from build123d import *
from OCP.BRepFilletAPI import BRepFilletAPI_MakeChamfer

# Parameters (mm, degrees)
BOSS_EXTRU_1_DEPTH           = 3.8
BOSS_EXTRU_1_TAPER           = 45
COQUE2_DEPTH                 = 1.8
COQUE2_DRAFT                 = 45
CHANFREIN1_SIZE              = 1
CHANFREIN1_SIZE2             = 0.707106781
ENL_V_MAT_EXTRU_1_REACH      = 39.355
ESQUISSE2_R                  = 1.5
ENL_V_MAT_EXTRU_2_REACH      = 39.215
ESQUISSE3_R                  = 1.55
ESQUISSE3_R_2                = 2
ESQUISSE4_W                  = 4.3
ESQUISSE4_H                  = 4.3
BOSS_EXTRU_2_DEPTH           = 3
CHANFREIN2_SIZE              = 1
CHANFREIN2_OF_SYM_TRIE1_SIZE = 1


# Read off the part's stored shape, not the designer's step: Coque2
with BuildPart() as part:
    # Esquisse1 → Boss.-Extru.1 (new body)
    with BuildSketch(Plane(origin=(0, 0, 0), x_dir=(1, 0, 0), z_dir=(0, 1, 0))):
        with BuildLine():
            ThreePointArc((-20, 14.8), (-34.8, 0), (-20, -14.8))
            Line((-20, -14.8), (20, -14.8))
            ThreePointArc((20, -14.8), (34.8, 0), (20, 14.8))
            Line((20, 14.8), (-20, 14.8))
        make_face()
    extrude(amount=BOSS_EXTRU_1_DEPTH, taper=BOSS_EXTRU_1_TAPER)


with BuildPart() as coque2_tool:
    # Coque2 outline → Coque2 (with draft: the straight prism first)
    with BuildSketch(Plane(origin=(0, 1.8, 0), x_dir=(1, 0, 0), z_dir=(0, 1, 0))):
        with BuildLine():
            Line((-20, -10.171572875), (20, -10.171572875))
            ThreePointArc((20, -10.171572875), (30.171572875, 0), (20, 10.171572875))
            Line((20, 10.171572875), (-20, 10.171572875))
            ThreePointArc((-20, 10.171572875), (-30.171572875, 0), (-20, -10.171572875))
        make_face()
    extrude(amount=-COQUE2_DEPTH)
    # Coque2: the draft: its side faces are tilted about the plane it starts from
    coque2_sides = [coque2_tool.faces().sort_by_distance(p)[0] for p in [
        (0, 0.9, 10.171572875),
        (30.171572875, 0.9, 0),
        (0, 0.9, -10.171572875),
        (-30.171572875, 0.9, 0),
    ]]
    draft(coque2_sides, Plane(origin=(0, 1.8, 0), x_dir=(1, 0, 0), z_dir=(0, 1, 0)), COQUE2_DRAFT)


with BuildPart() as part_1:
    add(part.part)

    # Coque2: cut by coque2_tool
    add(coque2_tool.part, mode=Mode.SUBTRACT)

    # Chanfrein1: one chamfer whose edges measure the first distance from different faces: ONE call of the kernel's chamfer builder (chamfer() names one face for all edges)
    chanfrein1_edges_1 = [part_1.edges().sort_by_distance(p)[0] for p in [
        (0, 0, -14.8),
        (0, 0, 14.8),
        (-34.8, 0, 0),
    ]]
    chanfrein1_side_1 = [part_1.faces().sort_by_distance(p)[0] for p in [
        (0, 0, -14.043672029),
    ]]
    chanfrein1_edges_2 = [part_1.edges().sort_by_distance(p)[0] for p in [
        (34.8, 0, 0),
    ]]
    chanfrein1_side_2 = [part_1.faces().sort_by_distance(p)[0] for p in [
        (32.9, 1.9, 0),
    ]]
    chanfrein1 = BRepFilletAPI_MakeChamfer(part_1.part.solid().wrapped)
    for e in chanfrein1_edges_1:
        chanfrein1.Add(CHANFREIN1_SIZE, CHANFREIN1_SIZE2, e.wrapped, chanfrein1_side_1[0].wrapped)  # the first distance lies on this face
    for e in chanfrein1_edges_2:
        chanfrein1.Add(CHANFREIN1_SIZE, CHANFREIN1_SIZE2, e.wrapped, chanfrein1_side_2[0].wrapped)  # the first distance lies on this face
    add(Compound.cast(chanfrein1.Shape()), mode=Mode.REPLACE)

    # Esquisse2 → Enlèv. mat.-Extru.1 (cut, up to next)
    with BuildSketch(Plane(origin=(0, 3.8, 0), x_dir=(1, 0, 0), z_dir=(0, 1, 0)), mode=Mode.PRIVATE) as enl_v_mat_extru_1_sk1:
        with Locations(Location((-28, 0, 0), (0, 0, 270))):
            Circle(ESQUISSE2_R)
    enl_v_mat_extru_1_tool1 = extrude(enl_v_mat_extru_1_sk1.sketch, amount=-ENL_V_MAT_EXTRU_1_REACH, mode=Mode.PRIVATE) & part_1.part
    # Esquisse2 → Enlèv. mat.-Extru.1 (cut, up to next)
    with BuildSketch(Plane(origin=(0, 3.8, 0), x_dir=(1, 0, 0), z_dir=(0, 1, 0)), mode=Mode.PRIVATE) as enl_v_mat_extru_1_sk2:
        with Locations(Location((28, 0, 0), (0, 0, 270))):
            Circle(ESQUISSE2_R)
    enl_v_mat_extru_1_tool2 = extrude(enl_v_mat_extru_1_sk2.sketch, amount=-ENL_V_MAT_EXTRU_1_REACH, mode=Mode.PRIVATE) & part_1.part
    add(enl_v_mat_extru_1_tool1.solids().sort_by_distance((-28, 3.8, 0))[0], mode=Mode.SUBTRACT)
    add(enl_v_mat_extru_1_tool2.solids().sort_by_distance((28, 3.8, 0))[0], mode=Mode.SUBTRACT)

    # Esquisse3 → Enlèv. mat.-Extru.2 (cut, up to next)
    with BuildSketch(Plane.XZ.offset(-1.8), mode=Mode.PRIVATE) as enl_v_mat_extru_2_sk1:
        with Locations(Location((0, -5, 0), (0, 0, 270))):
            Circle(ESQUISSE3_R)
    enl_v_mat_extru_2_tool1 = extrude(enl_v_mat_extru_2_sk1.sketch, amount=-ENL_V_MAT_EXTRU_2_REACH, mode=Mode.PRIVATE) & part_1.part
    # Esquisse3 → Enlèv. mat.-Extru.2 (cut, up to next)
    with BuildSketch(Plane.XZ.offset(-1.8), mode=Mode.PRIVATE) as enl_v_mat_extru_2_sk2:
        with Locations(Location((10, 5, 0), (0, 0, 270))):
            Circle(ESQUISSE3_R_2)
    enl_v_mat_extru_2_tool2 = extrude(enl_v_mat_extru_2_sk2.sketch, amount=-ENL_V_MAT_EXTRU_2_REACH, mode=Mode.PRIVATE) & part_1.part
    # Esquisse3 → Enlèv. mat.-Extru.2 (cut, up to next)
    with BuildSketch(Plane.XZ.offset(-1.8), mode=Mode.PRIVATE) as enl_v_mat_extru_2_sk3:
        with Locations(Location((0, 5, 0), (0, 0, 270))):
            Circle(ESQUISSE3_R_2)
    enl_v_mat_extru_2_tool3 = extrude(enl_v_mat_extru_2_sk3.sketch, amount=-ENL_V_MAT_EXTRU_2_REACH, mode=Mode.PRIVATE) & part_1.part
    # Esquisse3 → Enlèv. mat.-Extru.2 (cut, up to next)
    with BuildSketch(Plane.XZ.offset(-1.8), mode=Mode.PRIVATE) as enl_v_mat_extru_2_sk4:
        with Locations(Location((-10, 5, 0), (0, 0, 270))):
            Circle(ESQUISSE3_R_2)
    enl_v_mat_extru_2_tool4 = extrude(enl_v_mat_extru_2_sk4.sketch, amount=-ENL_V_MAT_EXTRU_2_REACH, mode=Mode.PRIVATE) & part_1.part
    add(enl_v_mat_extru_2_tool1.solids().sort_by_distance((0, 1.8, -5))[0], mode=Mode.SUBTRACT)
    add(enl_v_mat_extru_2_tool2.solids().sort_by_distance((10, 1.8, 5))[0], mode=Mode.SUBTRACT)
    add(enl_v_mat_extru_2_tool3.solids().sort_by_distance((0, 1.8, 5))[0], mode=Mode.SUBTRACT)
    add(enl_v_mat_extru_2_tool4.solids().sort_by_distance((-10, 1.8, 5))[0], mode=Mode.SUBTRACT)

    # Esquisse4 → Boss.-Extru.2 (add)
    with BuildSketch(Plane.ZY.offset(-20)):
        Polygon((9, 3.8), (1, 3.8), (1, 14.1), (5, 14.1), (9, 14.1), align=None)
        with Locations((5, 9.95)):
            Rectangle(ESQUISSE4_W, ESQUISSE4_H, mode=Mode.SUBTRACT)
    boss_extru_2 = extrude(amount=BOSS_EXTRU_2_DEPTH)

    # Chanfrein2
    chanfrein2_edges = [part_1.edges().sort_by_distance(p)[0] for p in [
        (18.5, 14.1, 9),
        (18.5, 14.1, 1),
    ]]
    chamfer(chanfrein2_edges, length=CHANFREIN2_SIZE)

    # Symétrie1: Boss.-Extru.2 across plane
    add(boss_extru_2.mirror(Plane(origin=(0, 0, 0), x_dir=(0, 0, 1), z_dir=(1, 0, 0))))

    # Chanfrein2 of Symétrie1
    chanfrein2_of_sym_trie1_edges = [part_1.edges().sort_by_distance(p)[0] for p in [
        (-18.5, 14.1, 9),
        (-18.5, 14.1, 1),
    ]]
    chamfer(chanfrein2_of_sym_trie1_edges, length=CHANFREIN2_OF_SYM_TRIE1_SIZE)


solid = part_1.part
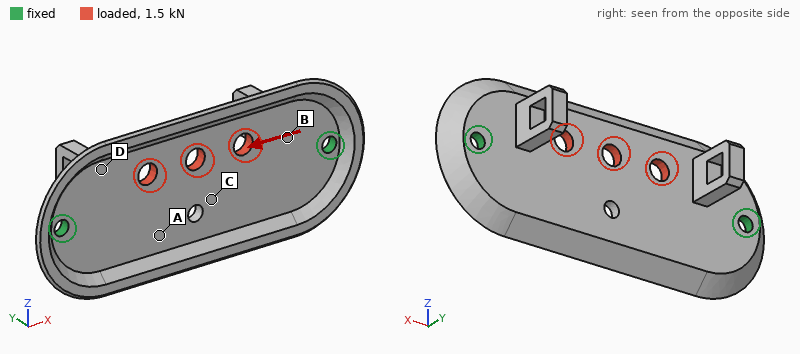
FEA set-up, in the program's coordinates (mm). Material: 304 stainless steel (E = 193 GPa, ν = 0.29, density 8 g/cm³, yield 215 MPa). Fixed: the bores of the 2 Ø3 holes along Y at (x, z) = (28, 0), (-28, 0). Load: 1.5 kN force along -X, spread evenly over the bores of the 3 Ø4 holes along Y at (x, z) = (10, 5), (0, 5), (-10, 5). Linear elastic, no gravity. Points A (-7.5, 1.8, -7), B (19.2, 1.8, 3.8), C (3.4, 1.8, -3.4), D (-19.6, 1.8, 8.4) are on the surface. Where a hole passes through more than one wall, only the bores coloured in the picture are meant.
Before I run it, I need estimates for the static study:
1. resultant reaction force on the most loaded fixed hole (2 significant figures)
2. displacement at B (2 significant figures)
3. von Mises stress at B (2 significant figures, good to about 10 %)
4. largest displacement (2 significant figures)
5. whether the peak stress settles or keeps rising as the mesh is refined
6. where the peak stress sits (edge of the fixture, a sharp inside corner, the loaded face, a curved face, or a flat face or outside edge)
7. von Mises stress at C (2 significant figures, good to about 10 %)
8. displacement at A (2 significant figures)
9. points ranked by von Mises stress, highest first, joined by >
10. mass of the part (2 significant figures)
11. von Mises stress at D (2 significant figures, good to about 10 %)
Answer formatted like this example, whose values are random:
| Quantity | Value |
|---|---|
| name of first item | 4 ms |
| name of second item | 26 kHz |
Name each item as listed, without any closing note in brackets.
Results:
| Quantity | Value |
|---|---|
| resultant reaction force on the most loaded fixed hole | 760 N |
| displacement at B | 1.7 µm |
| von Mises stress at B | 29 MPa |
| largest displacement | 3.8 µm |
| whether the peak stress settles or keeps rising as the mesh is refined | keeps rising |
| where the peak stress sits | edge of the fixture |
| von Mises stress at C | 10 MPa |
| displacement at A | 1.9 µm |
| points ranked by von Mises stress, highest first, joined by > | B > D > C > A |
| mass of the part | 31 g |
| von Mises stress at D | 19 MPa |
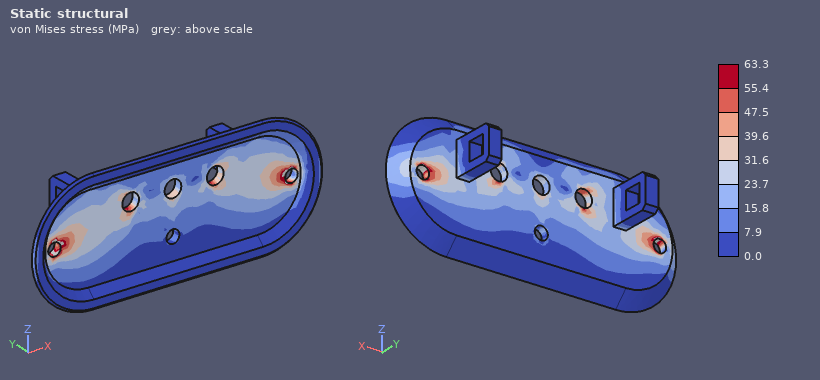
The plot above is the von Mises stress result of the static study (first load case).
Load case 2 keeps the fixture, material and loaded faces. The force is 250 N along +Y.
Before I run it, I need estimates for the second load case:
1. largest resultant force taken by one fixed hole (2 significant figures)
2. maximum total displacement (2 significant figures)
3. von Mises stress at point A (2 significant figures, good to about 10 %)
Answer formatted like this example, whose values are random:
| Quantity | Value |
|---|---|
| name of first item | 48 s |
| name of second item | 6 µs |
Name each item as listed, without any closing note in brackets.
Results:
| Quantity | Value |
|---|---|
| largest resultant force taken by one fixed hole | 180 N |
| maximum total displacement | 65 µm |
| von Mises stress at point A | 28 MPa |
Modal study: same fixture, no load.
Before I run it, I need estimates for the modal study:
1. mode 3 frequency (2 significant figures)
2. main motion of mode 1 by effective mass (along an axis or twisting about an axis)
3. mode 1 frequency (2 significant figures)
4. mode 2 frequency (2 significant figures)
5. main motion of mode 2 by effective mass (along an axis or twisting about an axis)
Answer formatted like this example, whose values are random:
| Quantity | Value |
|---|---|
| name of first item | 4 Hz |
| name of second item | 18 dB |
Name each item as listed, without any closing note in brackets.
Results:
| Quantity | Value |
|---|---|
| mode 3 frequency | 7500 Hz |
| main motion of mode 1 by effective mass | along Y |
| mode 1 frequency | 3400 Hz |
| mode 2 frequency | 3900 Hz |
| main motion of mode 2 by effective mass | twisting about X |
